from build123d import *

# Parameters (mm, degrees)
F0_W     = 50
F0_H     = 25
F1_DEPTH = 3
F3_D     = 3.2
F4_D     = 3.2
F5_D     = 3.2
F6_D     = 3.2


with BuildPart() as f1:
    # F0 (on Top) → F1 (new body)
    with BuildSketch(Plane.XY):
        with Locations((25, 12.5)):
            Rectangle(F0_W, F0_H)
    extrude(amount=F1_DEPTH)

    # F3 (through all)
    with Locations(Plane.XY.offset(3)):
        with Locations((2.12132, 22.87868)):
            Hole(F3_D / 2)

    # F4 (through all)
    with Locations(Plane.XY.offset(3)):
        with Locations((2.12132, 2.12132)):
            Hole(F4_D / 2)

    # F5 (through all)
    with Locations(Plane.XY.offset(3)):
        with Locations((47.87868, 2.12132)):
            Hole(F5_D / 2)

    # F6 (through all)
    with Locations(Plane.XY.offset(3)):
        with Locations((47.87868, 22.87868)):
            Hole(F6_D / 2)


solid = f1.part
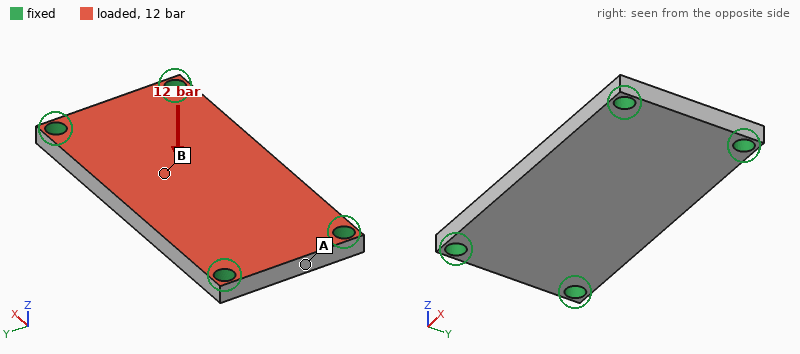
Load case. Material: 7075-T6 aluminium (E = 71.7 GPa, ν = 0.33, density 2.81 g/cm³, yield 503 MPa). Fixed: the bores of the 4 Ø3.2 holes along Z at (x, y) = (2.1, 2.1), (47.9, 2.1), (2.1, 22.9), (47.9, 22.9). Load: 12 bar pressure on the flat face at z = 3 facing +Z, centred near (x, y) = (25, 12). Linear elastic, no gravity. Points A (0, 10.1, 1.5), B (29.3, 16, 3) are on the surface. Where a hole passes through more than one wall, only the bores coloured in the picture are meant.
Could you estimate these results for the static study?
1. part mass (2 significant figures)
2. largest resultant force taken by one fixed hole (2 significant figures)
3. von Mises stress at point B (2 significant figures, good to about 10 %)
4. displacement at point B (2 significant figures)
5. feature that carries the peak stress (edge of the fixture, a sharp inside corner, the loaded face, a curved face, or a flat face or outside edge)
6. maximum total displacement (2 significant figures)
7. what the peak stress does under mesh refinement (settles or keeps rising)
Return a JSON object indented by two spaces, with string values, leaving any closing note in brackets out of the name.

{
  "part mass": "10 g",
  "largest resultant force taken by one fixed hole": "370 N",
  "von Mises stress at point B": "59 MPa",
  "displacement at point B": "0.091 mm",
  "feature that carries the peak stress": "edge of the fixture",
  "maximum total displacement": "0.10 mm",
  "what the peak stress does under mesh refinement": "keeps rising"
}
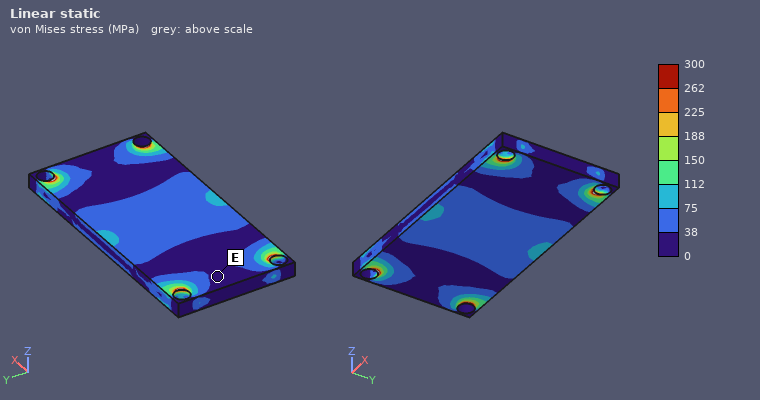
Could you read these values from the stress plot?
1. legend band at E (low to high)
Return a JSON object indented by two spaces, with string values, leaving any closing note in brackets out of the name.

{
  "legend band at E": "0 to 38 MPa"
}
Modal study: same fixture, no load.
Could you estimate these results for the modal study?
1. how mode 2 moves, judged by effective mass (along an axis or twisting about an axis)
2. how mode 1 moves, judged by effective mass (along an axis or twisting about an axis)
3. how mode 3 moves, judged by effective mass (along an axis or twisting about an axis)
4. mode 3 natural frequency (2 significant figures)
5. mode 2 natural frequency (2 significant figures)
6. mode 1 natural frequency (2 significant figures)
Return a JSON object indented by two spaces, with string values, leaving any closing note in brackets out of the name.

{
  "how mode 2 moves, judged by effective mass": "twisting about X",
  "how mode 1 moves, judged by effective mass": "along Z",
  "how mode 3 moves, judged by effective mass": "twisting about Y",
  "mode 3 natural frequency": "19 kHz",
  "mode 2 natural frequency": "12 kHz",
  "mode 1 natural frequency": "6900 Hz"
}
